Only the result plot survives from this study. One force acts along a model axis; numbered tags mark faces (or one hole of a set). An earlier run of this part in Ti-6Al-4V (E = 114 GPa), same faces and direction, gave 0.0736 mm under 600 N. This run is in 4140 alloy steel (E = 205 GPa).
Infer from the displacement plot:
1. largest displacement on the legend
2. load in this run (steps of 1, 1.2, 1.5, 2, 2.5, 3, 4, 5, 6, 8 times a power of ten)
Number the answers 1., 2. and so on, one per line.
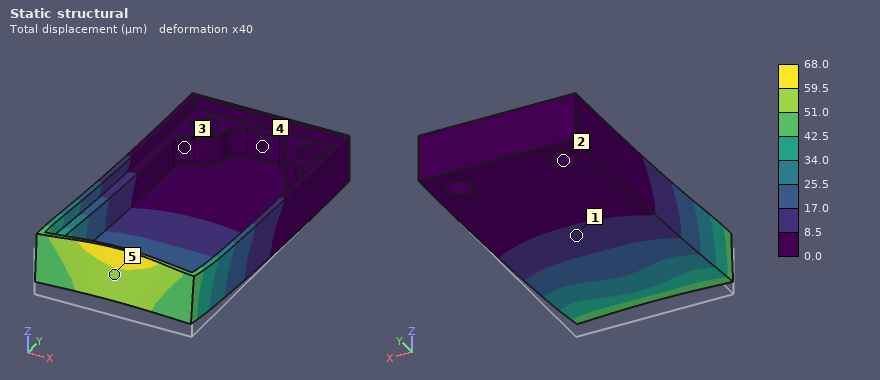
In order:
1. 68.0 µm
2. 1 kN
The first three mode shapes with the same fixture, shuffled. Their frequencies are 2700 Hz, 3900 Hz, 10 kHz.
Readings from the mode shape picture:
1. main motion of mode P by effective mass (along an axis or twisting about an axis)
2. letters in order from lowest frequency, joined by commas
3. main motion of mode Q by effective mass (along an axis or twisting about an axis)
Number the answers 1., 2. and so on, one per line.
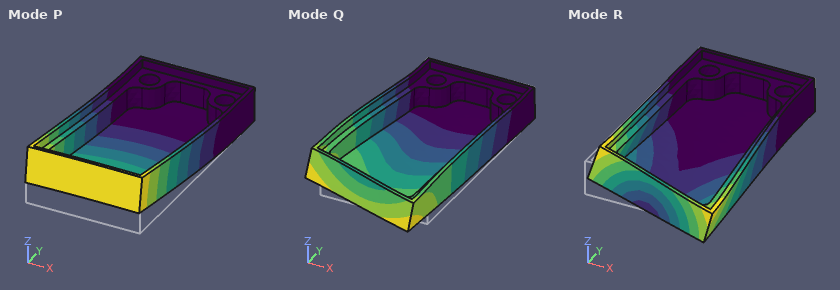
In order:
1. along Z
2. P, R, Q
3. along X
